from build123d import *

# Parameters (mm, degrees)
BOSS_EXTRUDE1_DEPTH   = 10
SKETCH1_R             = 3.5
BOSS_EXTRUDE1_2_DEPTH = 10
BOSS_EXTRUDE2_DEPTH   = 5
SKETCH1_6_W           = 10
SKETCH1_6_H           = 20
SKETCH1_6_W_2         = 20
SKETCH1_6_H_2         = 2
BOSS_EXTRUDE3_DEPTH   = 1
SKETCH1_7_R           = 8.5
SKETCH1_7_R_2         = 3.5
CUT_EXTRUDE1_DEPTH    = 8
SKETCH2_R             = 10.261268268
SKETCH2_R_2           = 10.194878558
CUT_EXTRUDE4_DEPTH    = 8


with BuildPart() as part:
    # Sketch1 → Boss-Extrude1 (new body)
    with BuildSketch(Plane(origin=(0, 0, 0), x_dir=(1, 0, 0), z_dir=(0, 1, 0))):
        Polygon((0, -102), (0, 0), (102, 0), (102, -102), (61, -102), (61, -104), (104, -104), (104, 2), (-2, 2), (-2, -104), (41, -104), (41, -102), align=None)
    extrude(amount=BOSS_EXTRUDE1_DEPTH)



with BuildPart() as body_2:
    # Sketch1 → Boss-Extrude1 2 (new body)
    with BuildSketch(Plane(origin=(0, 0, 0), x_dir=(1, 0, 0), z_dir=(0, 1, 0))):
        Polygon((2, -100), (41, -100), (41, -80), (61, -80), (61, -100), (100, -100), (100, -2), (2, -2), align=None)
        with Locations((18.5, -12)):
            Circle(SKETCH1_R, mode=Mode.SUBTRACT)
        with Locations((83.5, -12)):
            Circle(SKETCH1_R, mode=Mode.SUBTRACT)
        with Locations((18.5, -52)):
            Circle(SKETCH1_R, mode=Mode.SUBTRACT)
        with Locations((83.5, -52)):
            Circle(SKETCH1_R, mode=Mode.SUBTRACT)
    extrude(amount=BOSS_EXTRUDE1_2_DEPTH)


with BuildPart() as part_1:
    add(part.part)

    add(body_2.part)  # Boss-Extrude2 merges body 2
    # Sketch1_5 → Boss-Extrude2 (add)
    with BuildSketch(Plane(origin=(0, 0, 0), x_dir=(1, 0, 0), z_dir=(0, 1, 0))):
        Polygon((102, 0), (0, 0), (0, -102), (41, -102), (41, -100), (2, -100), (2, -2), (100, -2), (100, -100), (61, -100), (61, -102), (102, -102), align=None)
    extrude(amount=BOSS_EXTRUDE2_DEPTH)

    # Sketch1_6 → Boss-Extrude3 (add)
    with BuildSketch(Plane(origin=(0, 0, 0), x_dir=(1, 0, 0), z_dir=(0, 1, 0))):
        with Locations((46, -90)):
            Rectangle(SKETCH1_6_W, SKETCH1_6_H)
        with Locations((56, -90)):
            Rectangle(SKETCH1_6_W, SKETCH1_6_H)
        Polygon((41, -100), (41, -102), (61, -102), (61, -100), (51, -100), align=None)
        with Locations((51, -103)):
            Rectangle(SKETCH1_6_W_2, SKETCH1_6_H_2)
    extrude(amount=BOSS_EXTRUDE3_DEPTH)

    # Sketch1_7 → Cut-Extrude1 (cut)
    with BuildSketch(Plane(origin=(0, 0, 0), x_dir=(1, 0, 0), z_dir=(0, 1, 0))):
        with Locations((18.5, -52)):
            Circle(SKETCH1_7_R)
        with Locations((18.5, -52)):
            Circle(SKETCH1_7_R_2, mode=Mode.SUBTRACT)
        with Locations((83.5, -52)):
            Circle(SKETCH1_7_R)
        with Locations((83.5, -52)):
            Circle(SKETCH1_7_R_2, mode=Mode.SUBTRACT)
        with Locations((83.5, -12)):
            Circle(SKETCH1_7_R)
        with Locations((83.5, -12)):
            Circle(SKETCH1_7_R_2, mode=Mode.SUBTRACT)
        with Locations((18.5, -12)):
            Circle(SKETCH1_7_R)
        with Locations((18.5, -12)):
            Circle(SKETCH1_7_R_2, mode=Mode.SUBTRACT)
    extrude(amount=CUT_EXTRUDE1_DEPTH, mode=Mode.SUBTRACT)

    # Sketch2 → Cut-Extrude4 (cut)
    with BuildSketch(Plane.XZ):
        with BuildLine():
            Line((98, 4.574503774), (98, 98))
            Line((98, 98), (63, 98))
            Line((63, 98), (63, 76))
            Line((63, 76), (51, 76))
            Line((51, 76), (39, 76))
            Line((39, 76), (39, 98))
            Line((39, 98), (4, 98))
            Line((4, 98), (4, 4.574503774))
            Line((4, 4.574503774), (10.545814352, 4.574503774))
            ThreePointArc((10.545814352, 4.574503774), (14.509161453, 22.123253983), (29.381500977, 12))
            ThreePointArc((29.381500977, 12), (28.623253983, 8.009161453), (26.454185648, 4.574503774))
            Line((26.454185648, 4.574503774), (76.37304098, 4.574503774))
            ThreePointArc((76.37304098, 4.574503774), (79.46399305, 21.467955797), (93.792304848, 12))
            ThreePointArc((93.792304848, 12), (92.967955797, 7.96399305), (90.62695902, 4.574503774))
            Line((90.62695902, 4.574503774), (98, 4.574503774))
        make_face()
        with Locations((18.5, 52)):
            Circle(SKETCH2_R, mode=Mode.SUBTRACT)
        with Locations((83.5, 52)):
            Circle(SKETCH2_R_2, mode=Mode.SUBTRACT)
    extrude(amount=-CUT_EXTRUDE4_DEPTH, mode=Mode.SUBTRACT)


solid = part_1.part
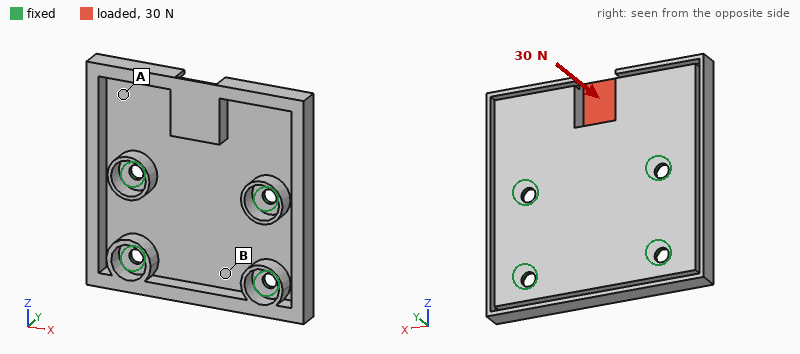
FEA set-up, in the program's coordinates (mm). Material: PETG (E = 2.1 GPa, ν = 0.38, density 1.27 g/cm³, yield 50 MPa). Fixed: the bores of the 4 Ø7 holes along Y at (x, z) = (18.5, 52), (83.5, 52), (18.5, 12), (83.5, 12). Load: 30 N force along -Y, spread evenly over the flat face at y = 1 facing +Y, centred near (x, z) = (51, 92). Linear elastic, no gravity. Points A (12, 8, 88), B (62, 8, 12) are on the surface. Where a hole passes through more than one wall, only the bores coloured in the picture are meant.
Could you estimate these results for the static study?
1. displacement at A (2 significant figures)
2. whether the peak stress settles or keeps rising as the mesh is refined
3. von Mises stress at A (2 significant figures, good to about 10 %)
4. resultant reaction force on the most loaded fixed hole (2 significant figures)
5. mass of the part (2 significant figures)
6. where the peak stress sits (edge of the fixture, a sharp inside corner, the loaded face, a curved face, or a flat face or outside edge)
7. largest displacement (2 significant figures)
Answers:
0.54 mm
keeps rising
0.95 MPa
40 N
52 g
edge of the fixture
1.4 mm
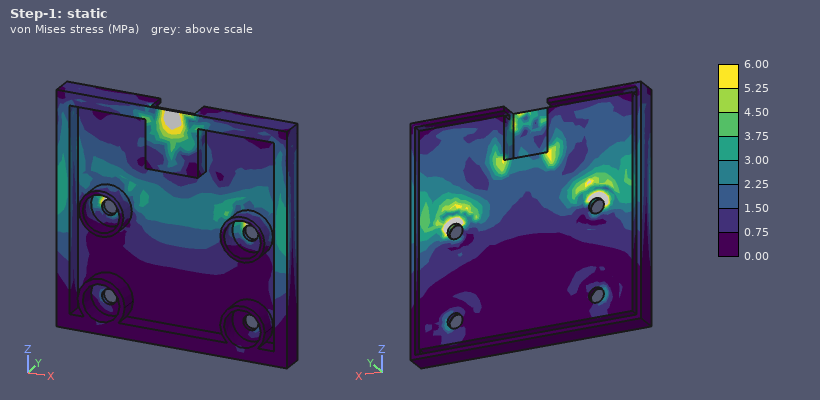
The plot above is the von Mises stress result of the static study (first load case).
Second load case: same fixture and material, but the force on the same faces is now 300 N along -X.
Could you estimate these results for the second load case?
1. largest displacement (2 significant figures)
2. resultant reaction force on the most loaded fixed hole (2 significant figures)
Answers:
1.6 mm
220 N
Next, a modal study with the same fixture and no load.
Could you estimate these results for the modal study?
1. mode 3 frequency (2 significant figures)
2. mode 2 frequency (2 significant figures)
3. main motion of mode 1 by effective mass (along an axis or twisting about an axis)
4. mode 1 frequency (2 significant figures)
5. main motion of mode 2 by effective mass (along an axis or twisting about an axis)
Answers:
700 Hz
380 Hz
along Y
270 Hz
twisting about Z
